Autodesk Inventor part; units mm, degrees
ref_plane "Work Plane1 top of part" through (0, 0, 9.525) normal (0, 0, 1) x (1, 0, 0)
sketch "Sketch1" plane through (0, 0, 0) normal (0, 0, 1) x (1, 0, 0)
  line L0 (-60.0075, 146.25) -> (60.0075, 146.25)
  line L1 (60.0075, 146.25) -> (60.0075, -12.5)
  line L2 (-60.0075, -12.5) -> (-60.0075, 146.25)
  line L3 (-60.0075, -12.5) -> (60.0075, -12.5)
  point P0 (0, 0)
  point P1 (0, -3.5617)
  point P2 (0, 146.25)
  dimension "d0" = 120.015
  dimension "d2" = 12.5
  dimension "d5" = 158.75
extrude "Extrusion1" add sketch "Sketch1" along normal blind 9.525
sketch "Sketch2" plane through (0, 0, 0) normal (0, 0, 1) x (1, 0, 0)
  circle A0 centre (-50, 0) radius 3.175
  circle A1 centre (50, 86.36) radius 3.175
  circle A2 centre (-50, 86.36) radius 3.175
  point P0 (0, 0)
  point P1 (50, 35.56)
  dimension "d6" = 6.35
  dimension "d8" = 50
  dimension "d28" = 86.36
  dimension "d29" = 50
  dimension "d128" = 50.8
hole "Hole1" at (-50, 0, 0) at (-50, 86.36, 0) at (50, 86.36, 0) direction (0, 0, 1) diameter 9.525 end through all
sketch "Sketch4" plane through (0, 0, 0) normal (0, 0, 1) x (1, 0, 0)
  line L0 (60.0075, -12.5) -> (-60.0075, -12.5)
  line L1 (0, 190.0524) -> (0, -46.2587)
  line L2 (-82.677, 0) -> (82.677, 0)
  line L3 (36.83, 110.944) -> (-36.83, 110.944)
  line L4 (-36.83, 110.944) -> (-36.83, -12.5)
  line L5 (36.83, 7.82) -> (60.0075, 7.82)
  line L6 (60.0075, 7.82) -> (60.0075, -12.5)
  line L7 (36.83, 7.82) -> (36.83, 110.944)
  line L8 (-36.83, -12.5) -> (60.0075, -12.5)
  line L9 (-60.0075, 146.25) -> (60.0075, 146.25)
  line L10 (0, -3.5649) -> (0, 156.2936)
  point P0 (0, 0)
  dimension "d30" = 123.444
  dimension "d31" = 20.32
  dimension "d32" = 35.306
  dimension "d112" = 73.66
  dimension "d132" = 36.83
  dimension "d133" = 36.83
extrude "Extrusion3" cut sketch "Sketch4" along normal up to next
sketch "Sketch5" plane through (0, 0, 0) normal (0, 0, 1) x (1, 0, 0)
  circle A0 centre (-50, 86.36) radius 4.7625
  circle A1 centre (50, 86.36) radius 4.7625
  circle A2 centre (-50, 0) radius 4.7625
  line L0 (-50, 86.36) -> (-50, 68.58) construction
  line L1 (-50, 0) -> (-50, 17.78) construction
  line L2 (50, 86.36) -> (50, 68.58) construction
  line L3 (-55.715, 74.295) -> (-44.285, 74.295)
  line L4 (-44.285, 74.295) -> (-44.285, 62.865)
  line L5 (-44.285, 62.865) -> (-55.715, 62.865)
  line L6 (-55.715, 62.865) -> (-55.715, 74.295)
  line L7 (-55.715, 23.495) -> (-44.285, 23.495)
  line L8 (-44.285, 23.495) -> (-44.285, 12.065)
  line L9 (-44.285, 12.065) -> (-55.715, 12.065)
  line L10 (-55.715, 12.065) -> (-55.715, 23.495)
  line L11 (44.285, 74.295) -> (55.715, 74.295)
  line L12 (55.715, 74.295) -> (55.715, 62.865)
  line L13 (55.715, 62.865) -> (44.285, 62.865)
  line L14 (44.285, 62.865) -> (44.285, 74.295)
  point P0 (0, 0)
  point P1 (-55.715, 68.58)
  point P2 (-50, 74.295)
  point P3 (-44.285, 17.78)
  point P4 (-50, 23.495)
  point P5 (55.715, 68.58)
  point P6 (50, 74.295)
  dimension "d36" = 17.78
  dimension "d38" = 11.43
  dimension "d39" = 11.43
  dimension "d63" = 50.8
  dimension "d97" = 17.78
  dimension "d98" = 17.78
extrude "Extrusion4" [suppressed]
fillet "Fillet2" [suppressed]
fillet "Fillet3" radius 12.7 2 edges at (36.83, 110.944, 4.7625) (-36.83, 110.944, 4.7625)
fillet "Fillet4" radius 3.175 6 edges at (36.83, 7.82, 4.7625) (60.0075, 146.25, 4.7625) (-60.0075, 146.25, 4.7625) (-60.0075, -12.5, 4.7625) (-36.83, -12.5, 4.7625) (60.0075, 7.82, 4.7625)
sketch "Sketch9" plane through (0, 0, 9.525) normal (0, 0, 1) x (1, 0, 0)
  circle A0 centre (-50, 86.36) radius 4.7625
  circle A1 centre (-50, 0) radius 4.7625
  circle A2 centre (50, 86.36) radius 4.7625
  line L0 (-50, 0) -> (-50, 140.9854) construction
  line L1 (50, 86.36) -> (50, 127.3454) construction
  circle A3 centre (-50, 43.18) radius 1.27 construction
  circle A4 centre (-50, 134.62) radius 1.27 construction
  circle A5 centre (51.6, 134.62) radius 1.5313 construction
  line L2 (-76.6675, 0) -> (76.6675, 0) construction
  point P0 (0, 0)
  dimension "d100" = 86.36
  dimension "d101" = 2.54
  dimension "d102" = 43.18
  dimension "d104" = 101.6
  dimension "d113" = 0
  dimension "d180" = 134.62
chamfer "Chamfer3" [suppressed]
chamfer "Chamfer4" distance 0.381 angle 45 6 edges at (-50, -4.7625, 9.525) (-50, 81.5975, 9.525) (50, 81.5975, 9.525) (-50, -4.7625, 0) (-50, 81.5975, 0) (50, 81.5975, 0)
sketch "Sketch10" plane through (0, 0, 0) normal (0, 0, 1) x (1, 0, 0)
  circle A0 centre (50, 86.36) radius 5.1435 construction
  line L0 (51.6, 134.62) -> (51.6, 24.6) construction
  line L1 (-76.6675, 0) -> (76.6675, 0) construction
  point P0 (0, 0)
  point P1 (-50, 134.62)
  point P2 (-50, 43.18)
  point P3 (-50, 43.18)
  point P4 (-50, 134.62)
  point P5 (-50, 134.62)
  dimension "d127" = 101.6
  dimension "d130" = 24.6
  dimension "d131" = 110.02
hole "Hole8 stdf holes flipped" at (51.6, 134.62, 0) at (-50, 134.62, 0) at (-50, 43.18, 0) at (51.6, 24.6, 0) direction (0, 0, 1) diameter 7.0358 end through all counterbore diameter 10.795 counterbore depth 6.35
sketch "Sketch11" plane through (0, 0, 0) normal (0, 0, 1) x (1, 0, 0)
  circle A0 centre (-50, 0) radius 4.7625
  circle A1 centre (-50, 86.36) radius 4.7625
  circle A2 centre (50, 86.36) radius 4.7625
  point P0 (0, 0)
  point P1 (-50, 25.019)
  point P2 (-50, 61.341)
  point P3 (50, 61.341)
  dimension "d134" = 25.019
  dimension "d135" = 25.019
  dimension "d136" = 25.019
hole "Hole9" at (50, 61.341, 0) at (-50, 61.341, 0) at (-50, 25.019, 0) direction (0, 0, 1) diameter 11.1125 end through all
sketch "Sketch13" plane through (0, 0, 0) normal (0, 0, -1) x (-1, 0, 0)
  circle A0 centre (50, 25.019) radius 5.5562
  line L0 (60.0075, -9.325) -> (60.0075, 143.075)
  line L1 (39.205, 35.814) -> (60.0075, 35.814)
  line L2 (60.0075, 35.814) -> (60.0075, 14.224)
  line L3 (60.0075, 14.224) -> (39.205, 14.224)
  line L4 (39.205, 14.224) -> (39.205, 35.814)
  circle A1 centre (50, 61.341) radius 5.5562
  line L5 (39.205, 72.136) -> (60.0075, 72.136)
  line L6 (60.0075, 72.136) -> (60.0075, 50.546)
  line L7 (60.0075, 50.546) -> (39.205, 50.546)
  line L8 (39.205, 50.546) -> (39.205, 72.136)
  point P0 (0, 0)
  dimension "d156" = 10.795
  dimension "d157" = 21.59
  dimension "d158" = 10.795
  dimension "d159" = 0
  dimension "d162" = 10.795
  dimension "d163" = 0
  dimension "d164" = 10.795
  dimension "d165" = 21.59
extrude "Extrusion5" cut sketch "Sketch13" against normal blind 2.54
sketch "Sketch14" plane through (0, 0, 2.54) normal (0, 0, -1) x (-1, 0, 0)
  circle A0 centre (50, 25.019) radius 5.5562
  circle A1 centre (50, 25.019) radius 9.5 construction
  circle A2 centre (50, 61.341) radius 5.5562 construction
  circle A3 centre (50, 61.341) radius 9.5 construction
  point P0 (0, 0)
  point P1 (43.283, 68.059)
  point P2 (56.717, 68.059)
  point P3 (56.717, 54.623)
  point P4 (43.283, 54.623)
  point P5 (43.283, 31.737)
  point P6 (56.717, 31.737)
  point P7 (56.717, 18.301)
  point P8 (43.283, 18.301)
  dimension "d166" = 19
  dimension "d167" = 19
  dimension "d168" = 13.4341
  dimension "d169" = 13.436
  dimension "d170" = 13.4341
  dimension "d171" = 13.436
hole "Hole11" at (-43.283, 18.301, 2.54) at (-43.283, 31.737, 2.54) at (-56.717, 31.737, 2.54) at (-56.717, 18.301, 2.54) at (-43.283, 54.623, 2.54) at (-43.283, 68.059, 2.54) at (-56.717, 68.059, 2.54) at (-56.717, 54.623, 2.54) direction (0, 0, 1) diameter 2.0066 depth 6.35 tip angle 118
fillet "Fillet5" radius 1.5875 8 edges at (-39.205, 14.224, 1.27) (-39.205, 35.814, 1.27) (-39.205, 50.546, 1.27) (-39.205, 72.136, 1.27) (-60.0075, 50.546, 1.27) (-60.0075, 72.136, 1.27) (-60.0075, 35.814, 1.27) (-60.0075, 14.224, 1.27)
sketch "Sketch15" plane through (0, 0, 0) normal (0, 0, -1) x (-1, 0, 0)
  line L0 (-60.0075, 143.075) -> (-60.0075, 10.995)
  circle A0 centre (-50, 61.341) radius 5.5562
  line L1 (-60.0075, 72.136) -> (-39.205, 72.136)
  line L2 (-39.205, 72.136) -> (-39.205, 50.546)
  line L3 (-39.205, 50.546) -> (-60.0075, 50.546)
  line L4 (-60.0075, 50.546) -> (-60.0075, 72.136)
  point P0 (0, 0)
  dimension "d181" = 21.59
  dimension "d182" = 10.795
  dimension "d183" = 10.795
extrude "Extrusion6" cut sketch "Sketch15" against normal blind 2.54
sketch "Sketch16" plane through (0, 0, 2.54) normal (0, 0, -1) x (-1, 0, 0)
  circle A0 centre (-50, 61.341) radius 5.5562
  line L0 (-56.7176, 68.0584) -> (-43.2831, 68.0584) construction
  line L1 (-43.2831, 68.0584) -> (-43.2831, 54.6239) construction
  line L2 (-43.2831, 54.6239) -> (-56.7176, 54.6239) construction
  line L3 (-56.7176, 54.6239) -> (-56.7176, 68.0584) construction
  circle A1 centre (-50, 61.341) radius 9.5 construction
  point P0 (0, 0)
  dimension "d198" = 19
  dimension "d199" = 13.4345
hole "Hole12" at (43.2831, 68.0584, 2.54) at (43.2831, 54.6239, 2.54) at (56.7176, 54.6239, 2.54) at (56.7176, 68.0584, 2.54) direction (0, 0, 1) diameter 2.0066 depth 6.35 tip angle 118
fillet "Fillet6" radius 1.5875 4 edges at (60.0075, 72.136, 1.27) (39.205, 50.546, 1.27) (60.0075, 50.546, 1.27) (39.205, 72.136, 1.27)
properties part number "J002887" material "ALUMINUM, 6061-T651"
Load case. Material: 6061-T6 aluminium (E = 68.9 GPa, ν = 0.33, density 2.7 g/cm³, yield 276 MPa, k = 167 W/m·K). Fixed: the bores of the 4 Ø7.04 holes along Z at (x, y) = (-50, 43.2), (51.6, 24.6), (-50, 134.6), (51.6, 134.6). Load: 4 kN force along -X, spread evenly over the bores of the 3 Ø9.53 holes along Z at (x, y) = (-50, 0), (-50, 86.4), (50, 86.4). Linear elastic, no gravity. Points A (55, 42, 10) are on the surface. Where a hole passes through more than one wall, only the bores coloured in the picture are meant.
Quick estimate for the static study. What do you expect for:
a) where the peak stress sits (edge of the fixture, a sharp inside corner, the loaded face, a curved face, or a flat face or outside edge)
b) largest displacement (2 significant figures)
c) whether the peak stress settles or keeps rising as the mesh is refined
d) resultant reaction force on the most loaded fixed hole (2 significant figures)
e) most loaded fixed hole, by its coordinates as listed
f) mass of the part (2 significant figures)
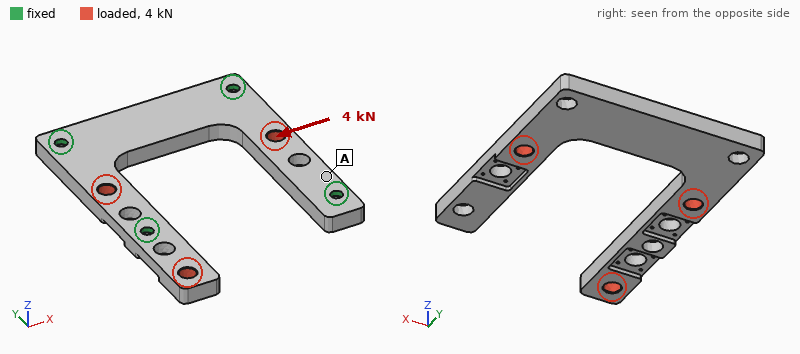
edge of the fixture
0.24 mm
keeps rising
2.3 kN
(-50, 43.2)
220 g
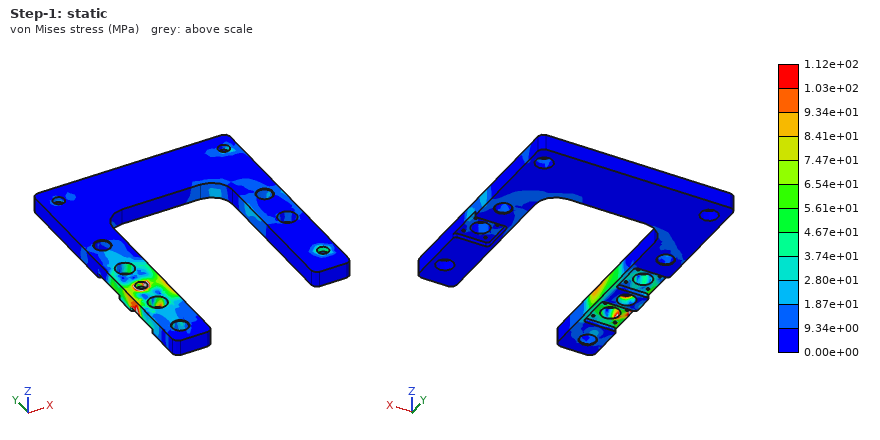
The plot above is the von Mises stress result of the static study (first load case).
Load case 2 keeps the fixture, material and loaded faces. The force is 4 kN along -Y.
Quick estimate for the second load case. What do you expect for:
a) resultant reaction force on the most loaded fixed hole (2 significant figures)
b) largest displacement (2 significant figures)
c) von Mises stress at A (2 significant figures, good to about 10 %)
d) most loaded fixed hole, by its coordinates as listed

1.7 kN
82 µm
6.0 MPa
(-50, 43.2)
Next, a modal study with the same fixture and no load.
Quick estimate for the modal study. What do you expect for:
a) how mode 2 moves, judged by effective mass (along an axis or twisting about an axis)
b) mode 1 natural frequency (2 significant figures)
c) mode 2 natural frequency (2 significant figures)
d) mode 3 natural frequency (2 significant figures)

along Z
1500 Hz
2800 Hz
3400 Hz
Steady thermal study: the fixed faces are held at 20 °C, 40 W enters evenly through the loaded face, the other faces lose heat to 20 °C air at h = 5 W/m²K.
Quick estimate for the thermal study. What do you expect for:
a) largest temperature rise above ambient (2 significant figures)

28 K
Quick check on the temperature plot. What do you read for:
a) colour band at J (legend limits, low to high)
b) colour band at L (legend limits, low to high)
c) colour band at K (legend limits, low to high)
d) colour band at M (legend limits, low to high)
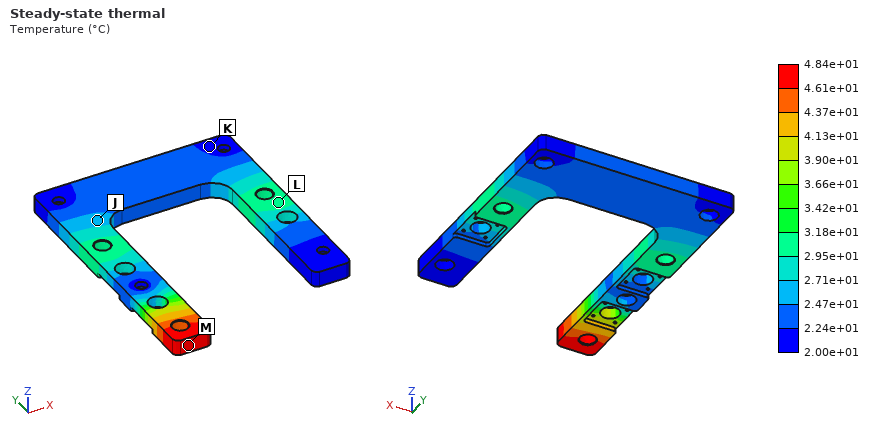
2.47e+01 to 2.71e+01 °C
2.95e+01 to 3.18e+01 °C
2.00e+01 to 2.24e+01 °C
4.61e+01 to 4.84e+01 °C
